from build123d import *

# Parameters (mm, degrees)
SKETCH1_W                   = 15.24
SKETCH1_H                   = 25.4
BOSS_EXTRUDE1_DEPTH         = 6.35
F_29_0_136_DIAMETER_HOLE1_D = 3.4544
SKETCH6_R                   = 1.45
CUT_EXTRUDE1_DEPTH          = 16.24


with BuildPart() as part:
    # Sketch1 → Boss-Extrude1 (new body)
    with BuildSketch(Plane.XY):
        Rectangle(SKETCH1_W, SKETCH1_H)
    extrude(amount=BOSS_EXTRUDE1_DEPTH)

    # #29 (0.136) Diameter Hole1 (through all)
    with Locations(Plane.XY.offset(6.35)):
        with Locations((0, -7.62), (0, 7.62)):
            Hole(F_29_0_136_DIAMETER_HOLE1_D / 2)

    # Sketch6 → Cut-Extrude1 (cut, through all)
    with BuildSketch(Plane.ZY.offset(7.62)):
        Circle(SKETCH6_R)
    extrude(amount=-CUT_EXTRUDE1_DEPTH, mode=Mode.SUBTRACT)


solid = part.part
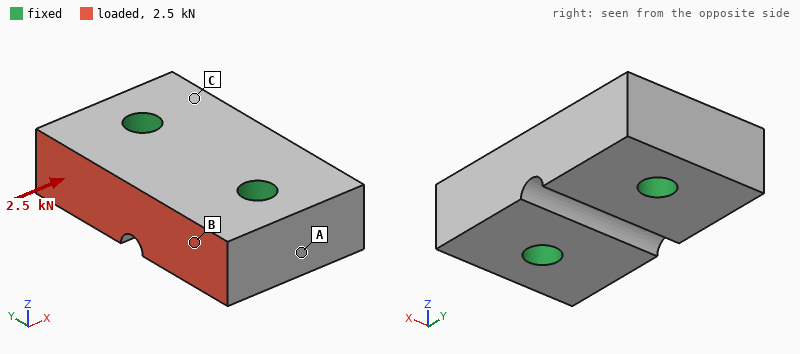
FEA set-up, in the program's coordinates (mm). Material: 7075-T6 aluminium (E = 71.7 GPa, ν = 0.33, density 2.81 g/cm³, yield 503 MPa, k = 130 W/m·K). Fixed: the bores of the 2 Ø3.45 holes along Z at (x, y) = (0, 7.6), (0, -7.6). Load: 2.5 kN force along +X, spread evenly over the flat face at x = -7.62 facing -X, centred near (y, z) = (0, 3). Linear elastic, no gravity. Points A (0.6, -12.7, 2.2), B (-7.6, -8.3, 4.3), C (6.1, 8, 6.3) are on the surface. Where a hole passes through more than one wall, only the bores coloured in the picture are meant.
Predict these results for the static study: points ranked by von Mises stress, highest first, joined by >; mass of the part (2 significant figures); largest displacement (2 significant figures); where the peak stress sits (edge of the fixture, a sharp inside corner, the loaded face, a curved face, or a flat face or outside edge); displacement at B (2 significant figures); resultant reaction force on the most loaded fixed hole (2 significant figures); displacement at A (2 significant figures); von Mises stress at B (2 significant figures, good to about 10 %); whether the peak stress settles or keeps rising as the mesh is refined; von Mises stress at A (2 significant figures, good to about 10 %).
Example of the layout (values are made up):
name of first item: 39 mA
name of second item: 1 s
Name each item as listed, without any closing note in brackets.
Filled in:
points ranked by von Mises stress, highest first, joined by >: B > A > C
mass of the part: 6.4 g
largest displacement: 2.5 µm
where the peak stress sits: edge of the fixture
displacement at B: 1.8 µm
resultant reaction force on the most loaded fixed hole: 1.3 kN
displacement at A: 0.67 µm
von Mises stress at B: 19 MPa
whether the peak stress settles or keeps rising as the mesh is refined: keeps rising
von Mises stress at A: 9.3 MPa
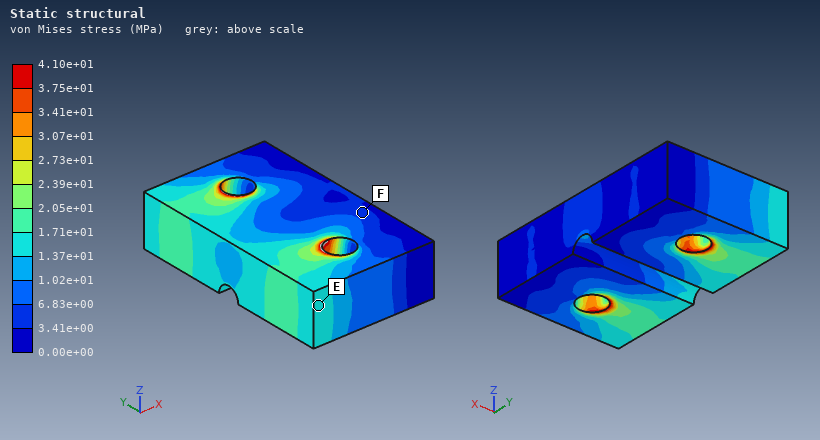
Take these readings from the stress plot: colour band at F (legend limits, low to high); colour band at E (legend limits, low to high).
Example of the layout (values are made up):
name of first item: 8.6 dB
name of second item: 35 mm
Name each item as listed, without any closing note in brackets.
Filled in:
colour band at F: 3.41e+00 to 6.83e+00 MPa
colour band at E: 1.37e+01 to 1.71e+01 MPa
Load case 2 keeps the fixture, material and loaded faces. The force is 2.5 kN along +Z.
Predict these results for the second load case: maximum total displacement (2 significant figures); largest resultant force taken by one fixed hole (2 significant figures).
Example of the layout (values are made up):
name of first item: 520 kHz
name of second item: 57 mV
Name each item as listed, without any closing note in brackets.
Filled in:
maximum total displacement: 19 µm
largest resultant force taken by one fixed hole: 1.3 kN
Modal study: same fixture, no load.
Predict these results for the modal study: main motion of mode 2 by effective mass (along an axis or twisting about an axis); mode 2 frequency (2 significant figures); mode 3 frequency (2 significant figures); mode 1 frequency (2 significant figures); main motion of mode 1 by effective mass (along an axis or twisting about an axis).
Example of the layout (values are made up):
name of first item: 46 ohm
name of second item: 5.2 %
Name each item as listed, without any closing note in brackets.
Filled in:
main motion of mode 2 by effective mass: along Z
mode 2 frequency: 64 kHz
mode 3 frequency: 72 kHz
mode 1 frequency: 56 kHz
main motion of mode 1 by effective mass: twisting about Y
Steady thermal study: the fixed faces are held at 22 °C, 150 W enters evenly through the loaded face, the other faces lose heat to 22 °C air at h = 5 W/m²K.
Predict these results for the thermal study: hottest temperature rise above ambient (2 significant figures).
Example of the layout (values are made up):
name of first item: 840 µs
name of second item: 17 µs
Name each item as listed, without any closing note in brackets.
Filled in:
hottest temperature rise above ambient: 59 K
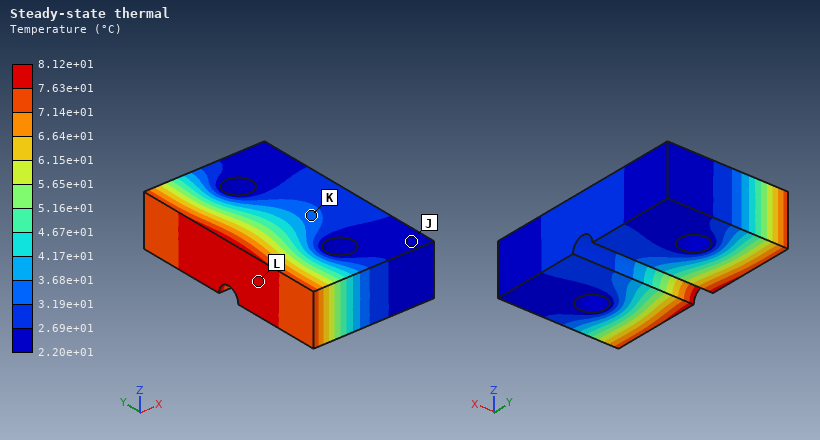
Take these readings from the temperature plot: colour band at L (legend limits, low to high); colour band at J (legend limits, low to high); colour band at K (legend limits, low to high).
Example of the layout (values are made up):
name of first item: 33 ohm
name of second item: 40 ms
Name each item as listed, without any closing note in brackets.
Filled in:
colour band at L: 7.63e+01 to 8.12e+01 °C
colour band at J: 2.20e+01 to 2.69e+01 °C
colour band at K: 3.19e+01 to 3.68e+01 °C
